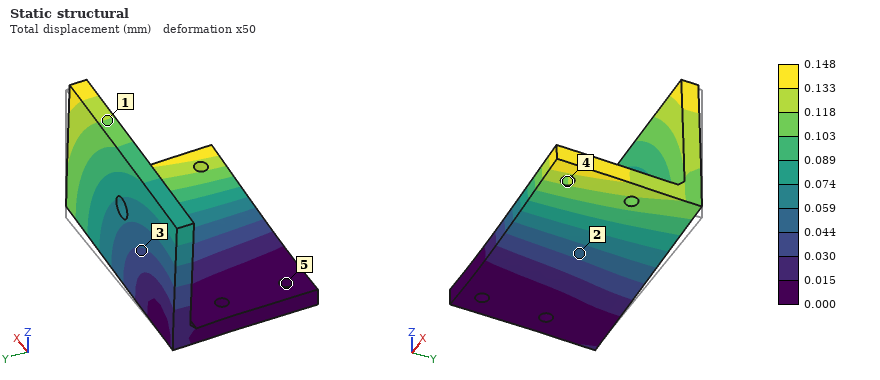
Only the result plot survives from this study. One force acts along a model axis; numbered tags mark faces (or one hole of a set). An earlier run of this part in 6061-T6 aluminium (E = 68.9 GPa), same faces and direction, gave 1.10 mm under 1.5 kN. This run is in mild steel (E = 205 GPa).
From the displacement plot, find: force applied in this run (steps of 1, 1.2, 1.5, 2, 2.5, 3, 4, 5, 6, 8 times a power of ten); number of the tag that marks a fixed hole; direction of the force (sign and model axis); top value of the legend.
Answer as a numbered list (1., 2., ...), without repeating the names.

1. 600 N
2. 5
3. +Z
4. 0.148 mm
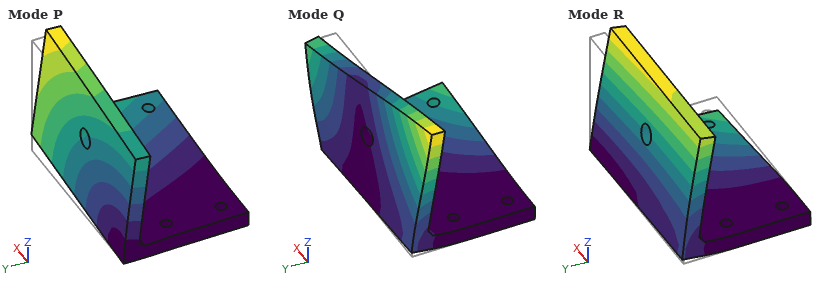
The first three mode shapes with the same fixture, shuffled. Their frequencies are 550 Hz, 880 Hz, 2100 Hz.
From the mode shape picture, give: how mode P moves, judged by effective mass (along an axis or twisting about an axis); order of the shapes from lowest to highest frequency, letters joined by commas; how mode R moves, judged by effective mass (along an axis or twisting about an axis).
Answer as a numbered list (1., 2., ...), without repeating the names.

1. along Z
2. P, R, Q
3. along Y
